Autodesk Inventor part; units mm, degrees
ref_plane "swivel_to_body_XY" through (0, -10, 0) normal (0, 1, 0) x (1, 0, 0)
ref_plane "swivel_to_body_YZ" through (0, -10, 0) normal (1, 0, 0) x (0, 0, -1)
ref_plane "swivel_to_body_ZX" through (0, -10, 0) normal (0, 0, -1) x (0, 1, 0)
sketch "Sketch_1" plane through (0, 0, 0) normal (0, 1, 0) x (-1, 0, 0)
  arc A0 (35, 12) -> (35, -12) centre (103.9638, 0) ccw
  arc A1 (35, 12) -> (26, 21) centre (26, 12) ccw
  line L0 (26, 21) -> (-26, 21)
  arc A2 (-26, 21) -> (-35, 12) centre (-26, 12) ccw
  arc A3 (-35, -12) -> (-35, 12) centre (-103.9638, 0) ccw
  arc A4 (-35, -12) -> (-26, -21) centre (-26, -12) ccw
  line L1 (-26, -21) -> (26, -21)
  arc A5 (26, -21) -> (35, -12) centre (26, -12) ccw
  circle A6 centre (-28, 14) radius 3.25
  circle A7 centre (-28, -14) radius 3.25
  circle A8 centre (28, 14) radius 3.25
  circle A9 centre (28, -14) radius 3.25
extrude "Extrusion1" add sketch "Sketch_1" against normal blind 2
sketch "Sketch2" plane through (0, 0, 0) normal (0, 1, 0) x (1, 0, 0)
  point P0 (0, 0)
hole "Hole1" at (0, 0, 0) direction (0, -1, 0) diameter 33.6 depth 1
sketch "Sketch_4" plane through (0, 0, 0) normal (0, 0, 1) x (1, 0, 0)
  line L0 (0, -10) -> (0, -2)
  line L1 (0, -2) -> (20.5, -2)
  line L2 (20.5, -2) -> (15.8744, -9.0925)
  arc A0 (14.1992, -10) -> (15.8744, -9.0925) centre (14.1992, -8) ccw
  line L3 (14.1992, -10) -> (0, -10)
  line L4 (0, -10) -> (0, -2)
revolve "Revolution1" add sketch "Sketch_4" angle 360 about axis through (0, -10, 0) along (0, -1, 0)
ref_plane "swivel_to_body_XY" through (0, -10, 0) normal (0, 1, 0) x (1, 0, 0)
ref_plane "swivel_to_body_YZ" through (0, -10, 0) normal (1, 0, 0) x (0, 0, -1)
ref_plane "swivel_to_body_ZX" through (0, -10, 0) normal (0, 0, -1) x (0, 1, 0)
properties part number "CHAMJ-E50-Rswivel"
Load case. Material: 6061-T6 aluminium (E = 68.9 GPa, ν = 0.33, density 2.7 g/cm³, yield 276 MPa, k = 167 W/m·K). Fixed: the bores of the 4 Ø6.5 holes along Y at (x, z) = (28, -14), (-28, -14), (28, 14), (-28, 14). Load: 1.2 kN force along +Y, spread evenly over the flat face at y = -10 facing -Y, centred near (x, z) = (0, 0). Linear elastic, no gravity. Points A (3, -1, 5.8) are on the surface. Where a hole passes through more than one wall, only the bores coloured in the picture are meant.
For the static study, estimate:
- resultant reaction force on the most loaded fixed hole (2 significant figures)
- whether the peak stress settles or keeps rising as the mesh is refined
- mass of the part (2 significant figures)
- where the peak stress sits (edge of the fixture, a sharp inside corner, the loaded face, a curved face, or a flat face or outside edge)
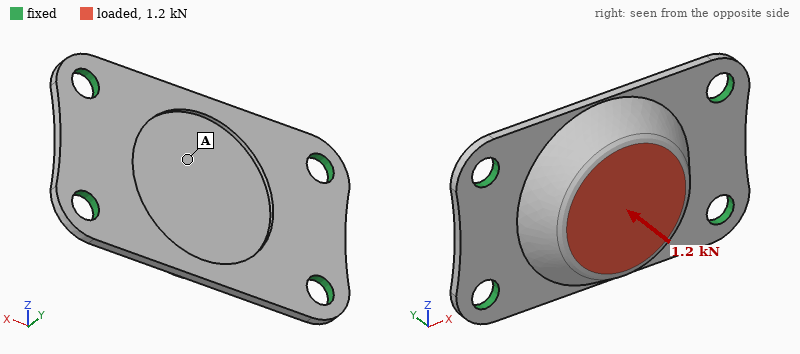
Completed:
500 N
keeps rising
34 g
edge of the fixture
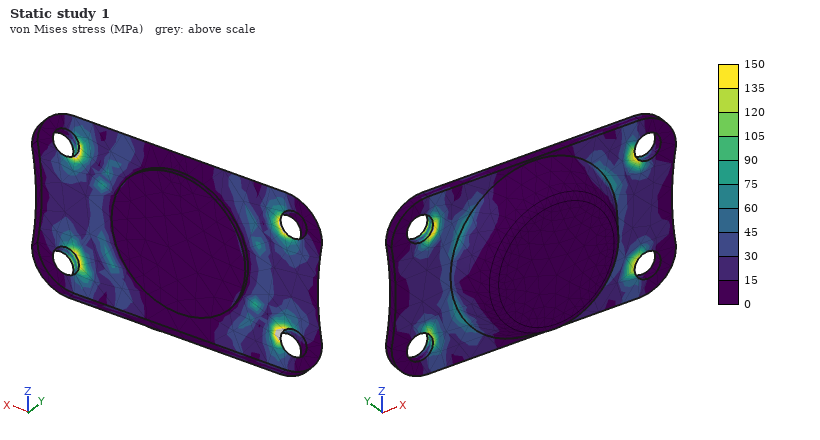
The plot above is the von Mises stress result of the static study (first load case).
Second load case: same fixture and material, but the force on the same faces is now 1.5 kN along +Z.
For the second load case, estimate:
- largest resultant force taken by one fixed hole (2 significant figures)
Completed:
600 N
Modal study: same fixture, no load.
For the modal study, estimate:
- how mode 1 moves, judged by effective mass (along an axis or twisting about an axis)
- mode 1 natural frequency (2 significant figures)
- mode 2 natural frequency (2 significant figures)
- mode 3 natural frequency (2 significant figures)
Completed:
along Y
5100 Hz
5700 Hz
11 kHz
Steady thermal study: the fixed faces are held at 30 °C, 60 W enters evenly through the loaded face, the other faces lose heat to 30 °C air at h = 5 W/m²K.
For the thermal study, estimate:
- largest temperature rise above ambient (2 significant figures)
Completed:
36 K
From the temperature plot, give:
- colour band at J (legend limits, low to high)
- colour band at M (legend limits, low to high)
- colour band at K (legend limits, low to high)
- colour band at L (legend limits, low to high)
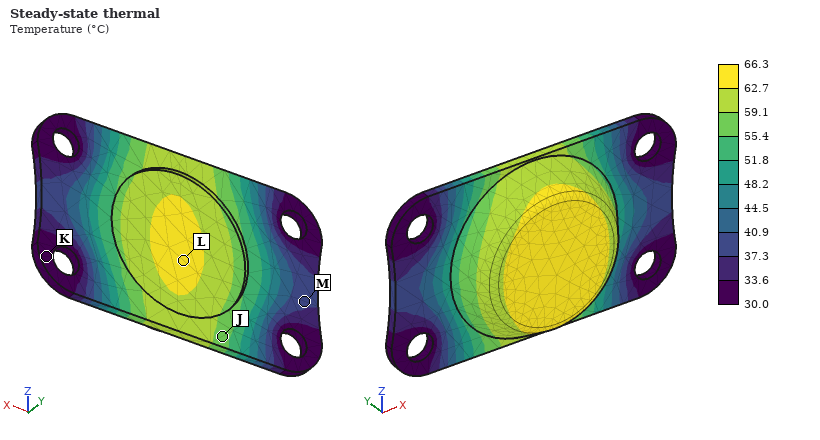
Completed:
55.4 to 59.1 °C
37.3 to 40.9 °C
30.0 to 33.6 °C
62.7 to 66.3 °C
